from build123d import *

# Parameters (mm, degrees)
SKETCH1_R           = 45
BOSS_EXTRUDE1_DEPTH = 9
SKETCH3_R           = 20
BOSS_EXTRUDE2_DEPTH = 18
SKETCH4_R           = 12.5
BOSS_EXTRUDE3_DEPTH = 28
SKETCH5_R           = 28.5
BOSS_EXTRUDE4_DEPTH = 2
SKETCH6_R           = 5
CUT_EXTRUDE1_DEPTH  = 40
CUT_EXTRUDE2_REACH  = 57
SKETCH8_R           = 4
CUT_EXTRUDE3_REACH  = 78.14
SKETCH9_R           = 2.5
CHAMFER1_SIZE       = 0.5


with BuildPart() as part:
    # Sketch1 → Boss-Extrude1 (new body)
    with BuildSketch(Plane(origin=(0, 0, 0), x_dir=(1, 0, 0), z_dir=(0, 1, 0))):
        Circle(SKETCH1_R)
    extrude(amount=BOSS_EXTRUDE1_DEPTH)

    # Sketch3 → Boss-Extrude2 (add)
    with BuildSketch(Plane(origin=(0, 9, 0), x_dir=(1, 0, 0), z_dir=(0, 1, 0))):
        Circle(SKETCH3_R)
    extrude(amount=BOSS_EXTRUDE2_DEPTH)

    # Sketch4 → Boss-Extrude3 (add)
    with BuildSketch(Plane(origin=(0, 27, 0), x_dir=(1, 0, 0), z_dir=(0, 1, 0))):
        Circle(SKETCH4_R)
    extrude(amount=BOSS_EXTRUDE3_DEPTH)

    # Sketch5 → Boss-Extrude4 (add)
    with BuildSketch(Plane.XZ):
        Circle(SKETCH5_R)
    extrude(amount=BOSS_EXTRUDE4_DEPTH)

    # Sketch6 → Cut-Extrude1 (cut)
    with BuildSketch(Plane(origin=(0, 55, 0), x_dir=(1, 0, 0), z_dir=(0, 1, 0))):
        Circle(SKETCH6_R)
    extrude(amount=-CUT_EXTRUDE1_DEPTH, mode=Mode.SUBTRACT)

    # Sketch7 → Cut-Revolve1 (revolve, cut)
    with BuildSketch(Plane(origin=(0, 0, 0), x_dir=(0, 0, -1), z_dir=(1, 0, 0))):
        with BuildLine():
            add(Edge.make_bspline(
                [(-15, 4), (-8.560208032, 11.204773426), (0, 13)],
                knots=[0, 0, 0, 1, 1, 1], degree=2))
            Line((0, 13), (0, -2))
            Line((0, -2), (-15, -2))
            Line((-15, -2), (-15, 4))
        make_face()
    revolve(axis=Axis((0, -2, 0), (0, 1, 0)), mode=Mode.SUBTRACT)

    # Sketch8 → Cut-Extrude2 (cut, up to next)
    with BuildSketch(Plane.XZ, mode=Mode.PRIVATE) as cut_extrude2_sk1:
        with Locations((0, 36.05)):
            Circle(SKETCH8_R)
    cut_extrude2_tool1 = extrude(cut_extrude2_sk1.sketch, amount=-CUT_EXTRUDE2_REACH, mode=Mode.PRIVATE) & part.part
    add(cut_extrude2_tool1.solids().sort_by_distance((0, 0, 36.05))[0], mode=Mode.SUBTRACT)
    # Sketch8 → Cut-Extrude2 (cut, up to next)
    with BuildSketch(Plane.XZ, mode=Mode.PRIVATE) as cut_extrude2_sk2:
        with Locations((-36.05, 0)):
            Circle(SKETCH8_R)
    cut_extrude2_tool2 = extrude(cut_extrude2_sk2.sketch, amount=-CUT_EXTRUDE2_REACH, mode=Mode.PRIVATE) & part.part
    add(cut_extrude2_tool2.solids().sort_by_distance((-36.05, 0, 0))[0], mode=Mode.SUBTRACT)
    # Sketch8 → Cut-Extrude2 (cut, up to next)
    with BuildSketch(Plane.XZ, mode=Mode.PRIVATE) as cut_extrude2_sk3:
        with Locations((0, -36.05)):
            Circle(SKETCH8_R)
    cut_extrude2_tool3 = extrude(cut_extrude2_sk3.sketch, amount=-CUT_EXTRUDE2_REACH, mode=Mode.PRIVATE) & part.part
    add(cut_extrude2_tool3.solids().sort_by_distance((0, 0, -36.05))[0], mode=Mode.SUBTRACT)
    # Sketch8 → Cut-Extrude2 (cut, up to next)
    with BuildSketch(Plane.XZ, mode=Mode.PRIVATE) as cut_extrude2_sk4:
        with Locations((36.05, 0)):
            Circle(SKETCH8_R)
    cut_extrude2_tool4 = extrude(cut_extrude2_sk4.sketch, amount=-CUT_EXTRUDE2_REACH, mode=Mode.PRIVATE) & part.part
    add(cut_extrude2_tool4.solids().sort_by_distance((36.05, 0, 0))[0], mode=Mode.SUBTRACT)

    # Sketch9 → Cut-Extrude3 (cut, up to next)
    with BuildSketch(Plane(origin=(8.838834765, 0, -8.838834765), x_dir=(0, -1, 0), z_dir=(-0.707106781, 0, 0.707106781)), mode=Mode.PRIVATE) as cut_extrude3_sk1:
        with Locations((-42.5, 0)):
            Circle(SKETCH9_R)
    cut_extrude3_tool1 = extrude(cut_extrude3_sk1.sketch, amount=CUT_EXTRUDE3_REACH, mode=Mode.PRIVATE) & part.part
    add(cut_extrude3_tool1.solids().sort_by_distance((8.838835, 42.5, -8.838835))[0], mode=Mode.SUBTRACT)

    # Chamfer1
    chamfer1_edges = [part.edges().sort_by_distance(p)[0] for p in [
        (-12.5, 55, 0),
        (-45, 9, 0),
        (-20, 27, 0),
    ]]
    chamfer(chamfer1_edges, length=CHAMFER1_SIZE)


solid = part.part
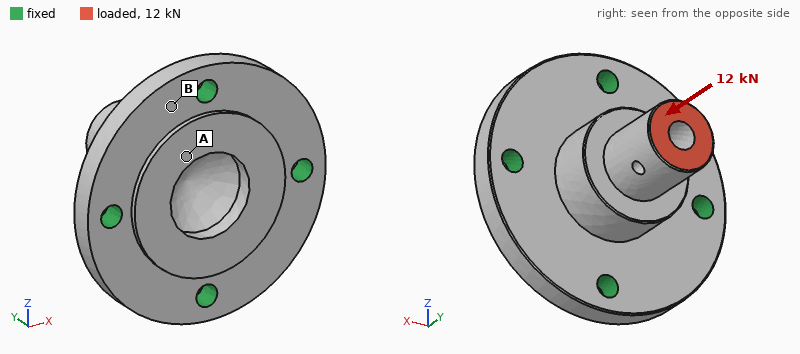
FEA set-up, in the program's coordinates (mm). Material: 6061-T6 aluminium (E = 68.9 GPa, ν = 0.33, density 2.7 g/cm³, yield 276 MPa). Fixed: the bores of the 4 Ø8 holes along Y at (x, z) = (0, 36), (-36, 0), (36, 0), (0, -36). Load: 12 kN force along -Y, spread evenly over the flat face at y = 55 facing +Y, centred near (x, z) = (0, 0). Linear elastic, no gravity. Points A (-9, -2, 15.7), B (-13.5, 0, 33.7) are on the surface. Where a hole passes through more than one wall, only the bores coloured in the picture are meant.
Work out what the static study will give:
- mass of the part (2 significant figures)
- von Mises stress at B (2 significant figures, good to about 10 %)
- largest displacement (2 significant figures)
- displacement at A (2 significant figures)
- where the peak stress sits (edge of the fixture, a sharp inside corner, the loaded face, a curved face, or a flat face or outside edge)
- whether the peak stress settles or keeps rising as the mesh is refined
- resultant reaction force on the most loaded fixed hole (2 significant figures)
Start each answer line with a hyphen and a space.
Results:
- 230 g
- 14 MPa
- 41 µm
- 22 µm
- edge of the fixture
- keeps rising
- 3.2 kN
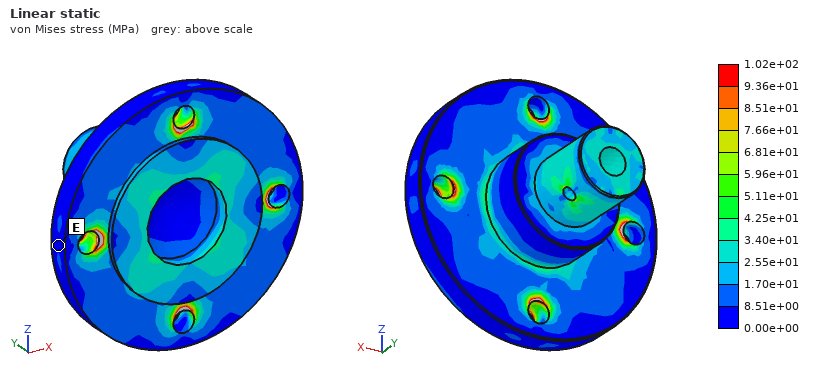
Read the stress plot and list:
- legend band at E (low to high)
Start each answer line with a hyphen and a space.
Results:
- 0.00e+00 to 8.51e+00 MPa
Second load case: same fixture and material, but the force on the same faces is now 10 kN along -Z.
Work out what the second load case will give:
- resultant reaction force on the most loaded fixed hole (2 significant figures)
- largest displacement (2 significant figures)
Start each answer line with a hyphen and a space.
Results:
- 8.7 kN
- 0.29 mm
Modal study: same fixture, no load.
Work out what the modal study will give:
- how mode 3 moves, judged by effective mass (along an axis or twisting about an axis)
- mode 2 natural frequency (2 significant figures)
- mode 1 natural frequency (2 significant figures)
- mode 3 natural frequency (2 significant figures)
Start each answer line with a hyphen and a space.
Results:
- along Y
- 7300 Hz
- 7200 Hz
- 9800 Hz
